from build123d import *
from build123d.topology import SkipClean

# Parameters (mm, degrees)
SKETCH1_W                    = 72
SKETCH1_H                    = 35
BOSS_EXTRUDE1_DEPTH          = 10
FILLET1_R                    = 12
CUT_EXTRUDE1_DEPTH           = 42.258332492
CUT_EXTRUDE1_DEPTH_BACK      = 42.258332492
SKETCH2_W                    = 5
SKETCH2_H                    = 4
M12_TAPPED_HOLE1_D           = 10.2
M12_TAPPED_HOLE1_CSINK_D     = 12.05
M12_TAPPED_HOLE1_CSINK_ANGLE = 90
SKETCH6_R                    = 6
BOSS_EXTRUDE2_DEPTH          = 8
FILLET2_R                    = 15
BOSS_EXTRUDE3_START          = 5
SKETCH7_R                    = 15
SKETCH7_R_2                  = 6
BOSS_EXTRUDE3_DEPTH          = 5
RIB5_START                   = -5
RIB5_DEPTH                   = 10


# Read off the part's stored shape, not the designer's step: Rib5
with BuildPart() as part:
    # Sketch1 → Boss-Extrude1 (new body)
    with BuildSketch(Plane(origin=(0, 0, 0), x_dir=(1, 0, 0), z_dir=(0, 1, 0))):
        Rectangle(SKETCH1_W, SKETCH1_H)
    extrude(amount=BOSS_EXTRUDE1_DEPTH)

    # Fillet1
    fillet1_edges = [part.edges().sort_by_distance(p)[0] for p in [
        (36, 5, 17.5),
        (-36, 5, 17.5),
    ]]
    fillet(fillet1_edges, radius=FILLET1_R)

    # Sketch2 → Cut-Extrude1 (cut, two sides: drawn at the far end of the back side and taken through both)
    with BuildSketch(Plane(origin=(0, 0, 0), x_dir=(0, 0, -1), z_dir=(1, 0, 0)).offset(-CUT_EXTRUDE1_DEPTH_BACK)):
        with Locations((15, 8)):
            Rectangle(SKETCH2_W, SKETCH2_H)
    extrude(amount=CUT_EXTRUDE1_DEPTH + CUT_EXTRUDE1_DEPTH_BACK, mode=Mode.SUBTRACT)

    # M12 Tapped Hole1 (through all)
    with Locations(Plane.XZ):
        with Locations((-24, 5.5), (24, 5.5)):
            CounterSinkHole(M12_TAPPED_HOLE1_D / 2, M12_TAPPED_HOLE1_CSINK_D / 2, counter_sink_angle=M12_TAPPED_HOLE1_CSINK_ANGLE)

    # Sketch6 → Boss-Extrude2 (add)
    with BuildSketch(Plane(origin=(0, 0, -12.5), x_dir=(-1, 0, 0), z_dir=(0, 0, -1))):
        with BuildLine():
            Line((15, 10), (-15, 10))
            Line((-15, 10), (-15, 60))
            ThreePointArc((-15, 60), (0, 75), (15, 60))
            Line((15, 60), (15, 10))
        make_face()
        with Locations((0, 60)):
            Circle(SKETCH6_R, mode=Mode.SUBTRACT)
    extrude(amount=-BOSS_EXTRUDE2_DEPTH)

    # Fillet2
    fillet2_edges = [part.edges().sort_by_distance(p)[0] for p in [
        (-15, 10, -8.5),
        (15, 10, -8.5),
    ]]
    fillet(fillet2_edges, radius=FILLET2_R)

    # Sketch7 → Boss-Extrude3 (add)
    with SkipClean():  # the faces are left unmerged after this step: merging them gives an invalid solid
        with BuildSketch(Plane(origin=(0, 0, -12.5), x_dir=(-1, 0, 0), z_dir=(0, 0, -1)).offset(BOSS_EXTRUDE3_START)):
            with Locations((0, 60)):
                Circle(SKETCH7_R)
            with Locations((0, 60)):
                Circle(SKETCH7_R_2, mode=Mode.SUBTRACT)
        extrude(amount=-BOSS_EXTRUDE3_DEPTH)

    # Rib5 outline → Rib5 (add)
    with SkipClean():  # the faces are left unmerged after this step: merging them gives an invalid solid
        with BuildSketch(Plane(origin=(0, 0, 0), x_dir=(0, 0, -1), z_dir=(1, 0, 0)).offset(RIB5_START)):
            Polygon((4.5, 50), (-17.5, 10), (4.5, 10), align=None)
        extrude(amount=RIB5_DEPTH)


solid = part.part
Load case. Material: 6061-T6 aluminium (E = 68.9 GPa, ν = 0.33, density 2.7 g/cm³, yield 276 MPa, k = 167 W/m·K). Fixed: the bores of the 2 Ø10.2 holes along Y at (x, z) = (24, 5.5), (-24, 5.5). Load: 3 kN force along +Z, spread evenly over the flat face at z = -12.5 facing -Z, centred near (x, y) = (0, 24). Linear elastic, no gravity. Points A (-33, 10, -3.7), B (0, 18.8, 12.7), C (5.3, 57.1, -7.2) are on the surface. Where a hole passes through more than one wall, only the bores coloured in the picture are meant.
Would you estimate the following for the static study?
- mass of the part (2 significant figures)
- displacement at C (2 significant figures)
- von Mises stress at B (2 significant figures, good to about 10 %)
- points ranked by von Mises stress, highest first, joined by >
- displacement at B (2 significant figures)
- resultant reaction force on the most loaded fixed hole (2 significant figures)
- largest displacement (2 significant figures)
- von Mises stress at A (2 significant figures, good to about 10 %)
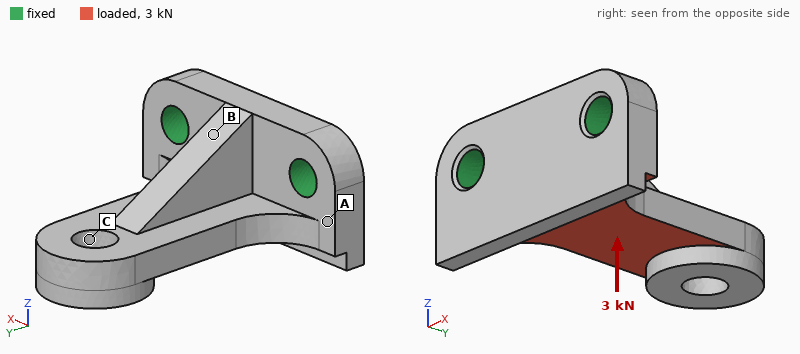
120 g
0.10 mm
24 MPa
B > A > C
0.031 mm
1.5 kN
0.14 mm
15 MPa
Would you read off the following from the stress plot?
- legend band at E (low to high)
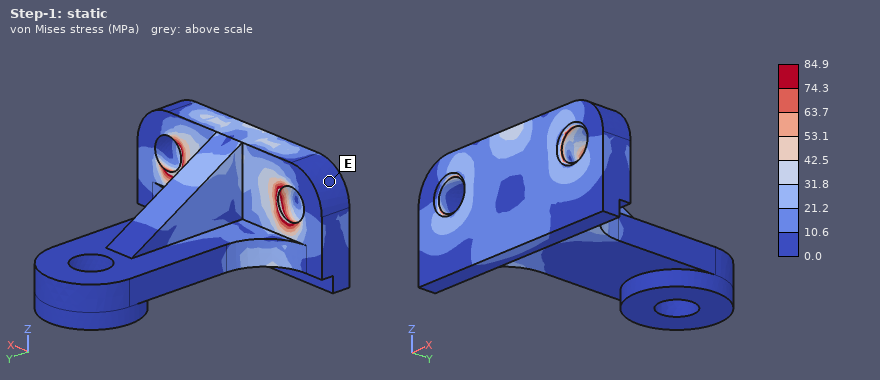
0.0 to 10.6 MPa
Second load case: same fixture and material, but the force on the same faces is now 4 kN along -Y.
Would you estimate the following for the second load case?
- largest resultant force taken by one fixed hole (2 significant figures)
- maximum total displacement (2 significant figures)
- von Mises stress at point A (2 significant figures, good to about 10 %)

2.0 kN
0.12 mm
19 MPa
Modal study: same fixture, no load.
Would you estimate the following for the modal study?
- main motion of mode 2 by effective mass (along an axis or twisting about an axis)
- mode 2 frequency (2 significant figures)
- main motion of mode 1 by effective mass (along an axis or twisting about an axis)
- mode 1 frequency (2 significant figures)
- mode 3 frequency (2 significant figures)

along X
4300 Hz
along Z
2500 Hz
7600 Hz
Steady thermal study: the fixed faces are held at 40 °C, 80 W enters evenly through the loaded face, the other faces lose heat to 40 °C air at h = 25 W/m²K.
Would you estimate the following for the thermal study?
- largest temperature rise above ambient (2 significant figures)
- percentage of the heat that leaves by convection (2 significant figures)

30 K
5.1 %
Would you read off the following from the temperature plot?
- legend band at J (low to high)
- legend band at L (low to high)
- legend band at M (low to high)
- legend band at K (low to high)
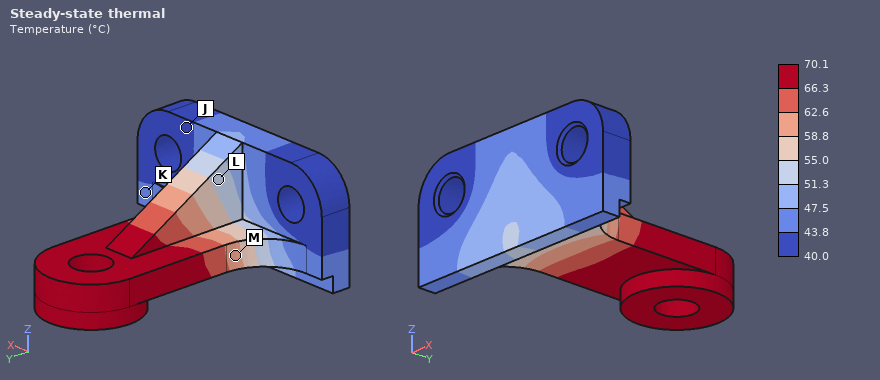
40.0 to 43.8 °C
51.3 to 55.0 °C
58.8 to 62.6 °C
43.8 to 47.5 °C
